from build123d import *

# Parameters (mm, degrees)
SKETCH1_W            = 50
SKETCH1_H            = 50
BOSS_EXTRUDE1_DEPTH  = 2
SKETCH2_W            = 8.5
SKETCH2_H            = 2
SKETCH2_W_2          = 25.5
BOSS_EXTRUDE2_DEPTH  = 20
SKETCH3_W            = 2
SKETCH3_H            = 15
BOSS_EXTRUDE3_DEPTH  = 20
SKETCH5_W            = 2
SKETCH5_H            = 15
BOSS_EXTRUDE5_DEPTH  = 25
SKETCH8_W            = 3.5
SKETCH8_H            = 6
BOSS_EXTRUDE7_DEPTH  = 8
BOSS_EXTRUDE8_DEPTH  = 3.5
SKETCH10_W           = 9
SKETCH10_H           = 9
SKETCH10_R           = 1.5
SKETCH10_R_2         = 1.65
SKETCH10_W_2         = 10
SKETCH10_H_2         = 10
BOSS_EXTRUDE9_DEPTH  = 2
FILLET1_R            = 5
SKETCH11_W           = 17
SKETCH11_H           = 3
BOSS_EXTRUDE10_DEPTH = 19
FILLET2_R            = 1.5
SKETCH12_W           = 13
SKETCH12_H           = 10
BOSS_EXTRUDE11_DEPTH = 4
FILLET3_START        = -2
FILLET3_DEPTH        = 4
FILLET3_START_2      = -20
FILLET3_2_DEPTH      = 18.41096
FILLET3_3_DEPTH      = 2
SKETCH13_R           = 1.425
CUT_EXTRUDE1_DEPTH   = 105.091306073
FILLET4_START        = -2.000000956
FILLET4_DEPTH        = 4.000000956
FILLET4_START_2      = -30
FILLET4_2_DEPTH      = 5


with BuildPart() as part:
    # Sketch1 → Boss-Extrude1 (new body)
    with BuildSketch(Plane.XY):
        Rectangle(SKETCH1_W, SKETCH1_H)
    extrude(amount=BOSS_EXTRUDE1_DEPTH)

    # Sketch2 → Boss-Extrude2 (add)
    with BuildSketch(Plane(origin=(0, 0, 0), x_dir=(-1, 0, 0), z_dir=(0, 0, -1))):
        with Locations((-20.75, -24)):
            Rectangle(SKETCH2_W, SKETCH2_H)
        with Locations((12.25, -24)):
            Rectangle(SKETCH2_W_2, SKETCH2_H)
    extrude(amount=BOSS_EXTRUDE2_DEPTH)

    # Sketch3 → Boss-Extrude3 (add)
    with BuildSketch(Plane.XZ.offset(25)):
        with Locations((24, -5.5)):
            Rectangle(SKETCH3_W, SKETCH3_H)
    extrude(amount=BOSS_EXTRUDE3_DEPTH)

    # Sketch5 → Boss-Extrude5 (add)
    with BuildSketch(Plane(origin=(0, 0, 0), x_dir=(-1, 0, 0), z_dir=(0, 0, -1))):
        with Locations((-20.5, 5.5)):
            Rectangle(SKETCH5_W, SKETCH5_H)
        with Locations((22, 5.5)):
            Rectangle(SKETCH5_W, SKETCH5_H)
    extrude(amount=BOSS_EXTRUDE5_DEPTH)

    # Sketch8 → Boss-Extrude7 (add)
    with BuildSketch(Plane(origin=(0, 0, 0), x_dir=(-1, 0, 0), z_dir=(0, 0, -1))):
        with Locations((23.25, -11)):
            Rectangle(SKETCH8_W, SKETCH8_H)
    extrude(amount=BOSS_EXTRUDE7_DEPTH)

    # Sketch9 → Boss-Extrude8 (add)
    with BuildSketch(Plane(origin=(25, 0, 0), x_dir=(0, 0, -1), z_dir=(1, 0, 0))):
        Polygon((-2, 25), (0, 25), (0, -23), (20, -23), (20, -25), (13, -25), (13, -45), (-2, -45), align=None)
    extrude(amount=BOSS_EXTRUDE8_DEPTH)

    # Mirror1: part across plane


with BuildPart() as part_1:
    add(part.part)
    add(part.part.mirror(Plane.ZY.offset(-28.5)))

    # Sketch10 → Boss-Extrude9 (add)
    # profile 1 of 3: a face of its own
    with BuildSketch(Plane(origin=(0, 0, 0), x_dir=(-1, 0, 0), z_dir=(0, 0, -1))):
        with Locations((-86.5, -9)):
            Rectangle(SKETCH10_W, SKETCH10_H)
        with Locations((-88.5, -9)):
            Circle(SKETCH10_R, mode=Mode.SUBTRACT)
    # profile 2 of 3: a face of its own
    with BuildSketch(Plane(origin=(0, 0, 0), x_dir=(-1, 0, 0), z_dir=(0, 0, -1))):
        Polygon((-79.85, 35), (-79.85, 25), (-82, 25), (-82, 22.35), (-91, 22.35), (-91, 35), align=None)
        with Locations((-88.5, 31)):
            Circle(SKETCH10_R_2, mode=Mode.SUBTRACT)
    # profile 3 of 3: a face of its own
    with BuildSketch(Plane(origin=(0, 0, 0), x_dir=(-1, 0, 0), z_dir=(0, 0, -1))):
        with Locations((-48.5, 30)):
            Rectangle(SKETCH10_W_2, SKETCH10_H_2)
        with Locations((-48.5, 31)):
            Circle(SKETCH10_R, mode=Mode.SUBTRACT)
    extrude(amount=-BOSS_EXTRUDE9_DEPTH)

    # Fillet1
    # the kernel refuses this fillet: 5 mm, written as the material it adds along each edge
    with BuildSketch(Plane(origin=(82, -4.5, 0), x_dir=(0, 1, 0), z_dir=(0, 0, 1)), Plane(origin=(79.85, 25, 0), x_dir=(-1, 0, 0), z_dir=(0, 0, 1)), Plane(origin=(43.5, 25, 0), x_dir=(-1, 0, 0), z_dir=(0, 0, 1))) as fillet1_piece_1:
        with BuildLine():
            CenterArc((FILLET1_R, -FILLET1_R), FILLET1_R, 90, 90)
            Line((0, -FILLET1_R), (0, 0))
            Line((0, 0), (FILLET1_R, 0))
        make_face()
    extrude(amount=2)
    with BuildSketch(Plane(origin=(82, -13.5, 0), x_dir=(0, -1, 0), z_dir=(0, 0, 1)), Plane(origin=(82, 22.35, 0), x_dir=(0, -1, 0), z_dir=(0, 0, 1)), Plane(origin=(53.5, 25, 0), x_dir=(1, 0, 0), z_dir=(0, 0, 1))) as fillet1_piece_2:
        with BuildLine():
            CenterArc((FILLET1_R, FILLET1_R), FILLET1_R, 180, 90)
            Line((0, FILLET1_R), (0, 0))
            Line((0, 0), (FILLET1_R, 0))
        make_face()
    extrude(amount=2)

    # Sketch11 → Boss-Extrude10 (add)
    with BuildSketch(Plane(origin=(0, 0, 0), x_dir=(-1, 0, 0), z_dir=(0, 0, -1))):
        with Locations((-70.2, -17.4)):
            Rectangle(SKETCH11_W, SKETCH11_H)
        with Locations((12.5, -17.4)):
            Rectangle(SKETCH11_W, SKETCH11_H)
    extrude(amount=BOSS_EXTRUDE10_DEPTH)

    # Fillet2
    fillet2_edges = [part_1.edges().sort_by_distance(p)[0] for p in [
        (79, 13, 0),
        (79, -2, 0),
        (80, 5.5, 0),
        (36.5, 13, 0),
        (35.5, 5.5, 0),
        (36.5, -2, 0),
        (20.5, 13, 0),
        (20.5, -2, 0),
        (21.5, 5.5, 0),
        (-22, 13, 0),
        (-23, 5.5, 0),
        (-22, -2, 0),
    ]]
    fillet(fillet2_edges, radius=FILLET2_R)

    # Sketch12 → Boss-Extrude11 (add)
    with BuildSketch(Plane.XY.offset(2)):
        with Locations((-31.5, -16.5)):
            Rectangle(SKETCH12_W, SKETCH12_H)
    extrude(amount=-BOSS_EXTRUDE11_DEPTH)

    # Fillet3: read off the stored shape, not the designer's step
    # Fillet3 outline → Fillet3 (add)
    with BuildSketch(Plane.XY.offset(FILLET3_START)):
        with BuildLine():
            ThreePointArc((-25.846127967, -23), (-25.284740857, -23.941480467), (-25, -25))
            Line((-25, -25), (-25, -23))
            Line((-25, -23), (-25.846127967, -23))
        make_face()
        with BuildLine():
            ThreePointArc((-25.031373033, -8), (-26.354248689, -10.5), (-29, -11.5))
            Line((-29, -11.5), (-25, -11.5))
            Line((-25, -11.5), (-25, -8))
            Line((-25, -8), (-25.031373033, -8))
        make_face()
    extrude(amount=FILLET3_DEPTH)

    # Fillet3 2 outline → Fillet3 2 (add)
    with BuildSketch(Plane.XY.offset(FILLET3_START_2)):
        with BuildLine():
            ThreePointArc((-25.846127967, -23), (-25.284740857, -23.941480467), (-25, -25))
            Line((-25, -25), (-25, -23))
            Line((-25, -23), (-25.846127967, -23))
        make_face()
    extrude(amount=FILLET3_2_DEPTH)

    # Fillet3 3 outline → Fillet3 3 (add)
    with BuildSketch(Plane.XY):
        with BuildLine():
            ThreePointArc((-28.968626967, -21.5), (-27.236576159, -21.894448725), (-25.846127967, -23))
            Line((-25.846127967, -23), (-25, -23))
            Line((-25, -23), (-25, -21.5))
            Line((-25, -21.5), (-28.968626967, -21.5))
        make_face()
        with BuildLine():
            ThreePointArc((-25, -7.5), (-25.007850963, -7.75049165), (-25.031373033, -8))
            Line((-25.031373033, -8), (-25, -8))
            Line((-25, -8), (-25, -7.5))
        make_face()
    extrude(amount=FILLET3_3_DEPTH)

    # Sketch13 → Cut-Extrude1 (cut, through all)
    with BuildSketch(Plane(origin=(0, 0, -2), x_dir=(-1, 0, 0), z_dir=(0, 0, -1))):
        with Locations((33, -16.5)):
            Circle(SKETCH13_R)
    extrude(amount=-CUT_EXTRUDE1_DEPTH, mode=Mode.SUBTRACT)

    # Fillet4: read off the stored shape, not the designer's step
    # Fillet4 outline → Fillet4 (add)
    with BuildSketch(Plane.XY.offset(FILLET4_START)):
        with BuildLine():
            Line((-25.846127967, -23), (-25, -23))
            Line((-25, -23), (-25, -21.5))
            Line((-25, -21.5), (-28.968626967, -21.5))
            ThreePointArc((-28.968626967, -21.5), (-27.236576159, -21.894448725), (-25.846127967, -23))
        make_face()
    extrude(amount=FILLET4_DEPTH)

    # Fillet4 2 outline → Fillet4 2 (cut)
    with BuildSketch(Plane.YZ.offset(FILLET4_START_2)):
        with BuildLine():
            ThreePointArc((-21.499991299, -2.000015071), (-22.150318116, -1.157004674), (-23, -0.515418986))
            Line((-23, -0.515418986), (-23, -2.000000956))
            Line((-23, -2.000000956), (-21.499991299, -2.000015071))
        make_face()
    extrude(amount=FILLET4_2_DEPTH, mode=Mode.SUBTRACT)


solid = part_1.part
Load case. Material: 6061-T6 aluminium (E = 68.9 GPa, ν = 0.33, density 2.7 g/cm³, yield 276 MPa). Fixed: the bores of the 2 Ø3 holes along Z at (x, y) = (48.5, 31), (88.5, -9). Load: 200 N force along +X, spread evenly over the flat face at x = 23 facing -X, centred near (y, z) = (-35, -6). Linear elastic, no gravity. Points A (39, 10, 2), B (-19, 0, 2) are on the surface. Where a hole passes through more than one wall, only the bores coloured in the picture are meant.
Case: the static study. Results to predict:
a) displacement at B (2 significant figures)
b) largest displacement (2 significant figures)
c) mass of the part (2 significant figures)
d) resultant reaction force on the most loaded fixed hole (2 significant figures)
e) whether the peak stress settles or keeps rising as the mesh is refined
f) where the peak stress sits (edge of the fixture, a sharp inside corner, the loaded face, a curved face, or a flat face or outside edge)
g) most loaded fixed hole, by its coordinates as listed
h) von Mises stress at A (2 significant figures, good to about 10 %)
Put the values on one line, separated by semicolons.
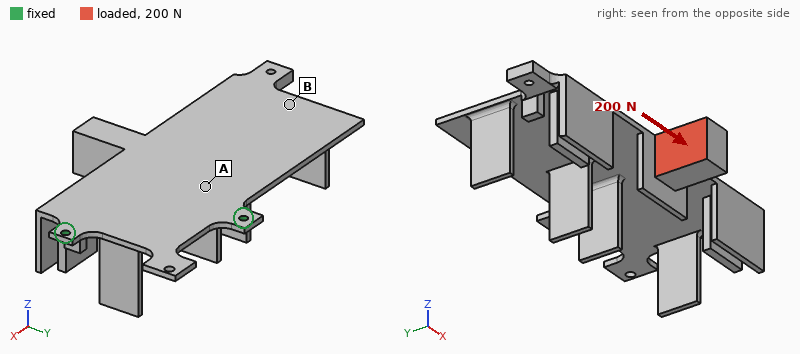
1.2 mm; 1.8 mm; 63 g; 260 N; keeps rising; edge of the fixture; (88.5, -9); 33 MPa
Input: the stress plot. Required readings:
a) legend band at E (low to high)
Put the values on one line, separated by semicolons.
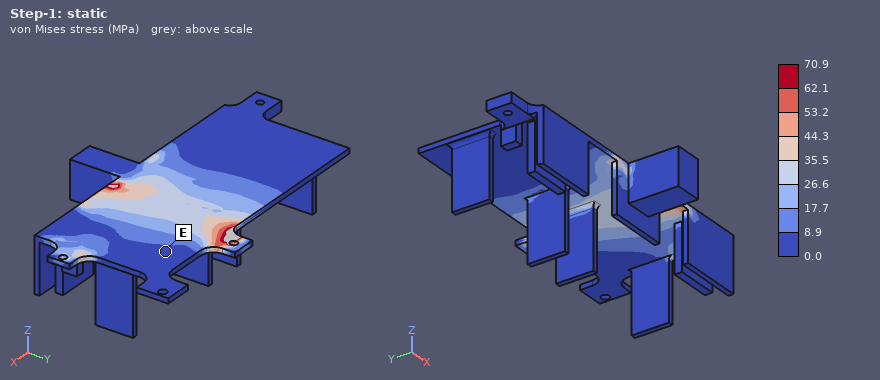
0.0 to 8.9 MPa
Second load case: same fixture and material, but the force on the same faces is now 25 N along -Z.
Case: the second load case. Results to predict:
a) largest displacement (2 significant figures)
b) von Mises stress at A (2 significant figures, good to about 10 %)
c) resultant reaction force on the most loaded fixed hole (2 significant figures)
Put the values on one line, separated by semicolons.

1.8 mm; 23 MPa; 13 N
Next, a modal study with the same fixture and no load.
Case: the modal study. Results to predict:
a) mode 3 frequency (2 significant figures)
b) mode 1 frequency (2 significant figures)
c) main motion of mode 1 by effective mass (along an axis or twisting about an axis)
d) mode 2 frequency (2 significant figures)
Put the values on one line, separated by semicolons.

700 Hz; 110 Hz; along Z; 340 Hz
